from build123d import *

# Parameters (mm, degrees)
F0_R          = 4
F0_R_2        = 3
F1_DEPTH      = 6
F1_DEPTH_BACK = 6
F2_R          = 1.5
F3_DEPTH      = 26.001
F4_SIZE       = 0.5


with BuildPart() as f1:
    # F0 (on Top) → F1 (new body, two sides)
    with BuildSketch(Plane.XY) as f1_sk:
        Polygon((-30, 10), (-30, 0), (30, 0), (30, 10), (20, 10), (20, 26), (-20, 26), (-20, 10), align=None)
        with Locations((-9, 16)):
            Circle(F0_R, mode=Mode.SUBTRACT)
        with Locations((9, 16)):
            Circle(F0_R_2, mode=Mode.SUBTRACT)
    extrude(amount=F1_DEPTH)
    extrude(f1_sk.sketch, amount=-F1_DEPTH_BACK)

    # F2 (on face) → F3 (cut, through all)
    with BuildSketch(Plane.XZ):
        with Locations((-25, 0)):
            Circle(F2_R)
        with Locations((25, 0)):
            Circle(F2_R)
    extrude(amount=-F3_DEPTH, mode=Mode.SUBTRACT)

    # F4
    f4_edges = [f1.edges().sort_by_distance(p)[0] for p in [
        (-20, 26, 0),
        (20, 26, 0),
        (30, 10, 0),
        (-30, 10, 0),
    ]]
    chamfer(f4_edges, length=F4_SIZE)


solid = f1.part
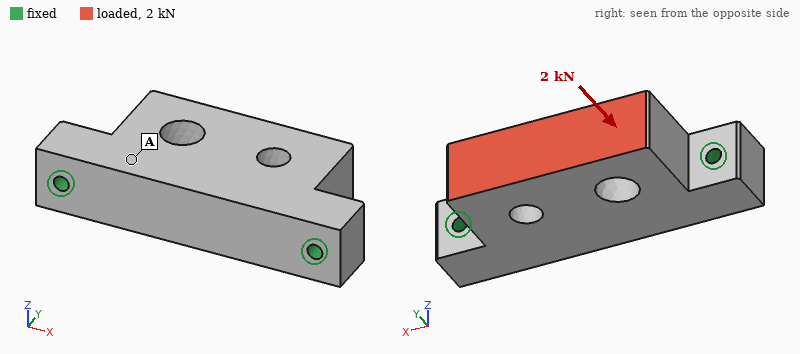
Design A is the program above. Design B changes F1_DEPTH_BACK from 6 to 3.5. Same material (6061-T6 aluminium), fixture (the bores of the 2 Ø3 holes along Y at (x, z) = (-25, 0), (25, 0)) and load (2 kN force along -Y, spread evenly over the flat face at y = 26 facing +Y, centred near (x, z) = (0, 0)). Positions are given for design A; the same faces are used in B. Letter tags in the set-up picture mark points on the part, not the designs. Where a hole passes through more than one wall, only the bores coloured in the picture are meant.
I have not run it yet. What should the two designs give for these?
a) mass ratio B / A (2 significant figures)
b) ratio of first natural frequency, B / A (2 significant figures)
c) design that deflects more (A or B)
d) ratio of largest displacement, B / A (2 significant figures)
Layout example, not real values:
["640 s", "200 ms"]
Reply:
["0.79", "0.92", "B", "1.3"]
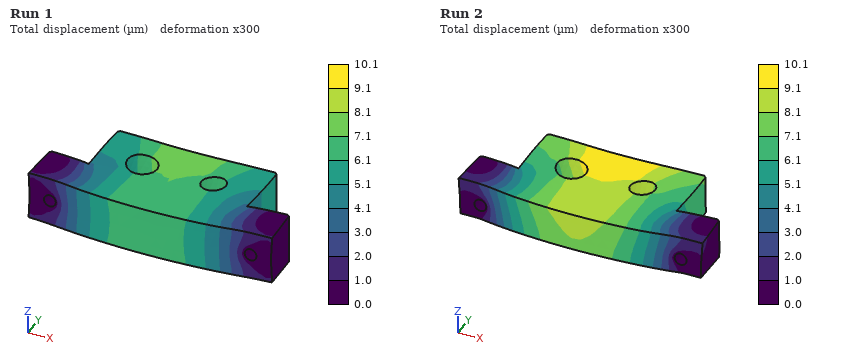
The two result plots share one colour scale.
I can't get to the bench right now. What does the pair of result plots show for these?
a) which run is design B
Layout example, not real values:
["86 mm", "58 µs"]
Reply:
["Run 2"]
